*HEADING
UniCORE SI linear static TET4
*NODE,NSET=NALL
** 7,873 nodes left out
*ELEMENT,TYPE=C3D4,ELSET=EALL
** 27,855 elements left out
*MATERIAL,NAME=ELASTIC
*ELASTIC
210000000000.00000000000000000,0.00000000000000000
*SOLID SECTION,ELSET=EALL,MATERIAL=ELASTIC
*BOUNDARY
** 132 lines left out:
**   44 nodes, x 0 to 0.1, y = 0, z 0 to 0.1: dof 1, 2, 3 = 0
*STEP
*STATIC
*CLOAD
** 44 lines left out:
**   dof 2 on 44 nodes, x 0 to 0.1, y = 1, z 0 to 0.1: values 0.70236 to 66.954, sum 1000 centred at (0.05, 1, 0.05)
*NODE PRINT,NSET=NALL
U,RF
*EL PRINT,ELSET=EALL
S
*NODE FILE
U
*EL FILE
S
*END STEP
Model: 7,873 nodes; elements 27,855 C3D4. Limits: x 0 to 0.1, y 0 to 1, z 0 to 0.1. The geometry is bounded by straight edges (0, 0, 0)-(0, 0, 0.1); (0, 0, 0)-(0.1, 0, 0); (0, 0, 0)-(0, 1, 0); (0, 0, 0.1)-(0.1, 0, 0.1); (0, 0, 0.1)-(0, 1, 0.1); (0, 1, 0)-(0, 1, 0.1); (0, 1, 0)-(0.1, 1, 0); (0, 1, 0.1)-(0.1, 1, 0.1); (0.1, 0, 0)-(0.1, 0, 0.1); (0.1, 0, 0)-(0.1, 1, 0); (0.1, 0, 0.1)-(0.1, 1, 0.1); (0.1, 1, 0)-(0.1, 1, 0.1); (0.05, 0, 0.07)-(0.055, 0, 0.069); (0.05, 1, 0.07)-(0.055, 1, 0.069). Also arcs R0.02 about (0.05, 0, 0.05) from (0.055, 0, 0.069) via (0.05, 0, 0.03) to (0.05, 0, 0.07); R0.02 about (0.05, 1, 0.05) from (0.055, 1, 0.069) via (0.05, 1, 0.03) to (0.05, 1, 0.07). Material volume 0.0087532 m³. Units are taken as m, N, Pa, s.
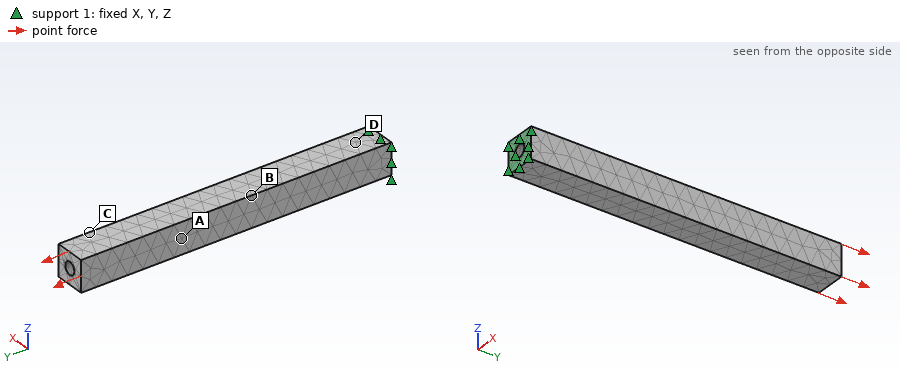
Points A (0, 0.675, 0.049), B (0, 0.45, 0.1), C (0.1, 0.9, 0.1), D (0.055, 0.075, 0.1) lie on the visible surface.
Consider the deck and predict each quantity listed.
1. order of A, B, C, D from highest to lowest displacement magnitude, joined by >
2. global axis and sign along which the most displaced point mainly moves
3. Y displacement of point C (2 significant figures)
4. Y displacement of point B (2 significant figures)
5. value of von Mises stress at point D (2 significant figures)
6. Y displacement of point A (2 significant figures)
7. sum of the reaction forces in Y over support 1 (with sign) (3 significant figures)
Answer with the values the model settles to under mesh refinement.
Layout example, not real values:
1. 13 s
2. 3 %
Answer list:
1. C > A > B > D
2. +Y
3. 4.9e-07 m
4. 2.4e-07 m
5. 1.1e+05 Pa
6. 3.7e-07 m
7. -1000 N
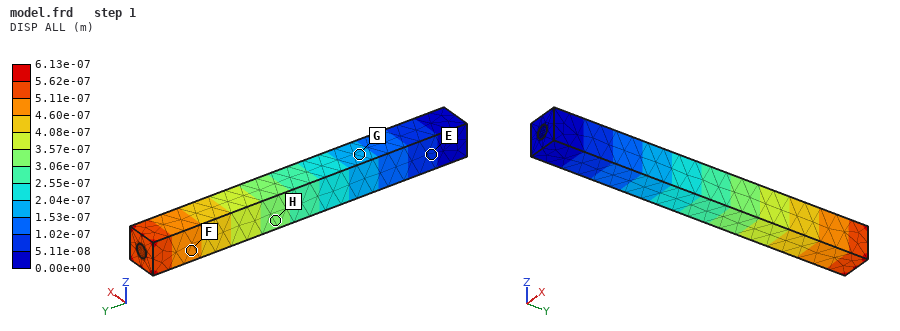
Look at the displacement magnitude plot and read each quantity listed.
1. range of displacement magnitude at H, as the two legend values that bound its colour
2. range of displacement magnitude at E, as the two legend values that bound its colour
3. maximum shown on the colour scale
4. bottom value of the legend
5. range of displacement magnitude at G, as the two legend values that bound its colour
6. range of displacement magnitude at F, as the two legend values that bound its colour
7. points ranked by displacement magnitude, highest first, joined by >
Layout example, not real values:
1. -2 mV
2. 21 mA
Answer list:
1. 3.06e-07 to 3.57e-07 m
2. 5.11e-08 to 1.02e-07 m
3. 6.13e-07 m
4. 0.00e+00 m
5. 1.53e-07 to 2.04e-07 m
6. 4.60e-07 to 5.11e-07 m
7. F > H > G > E
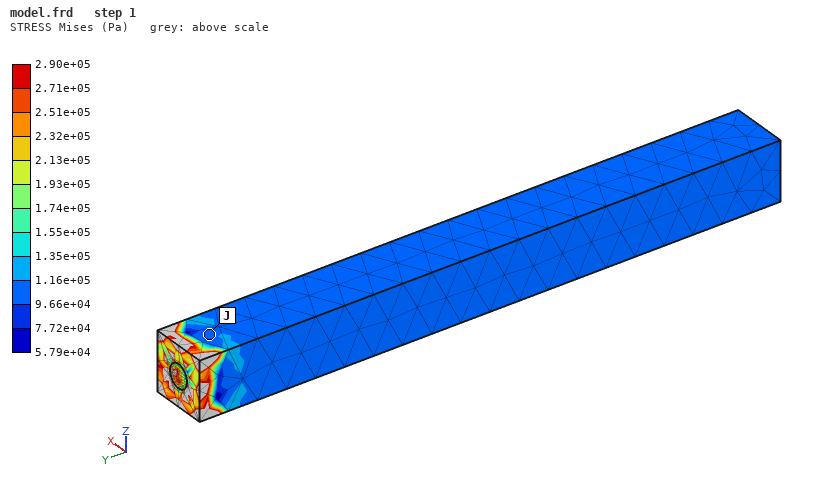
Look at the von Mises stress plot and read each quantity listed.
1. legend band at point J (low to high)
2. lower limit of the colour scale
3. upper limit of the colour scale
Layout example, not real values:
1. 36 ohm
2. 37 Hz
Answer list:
1. 9.66e+04 to 1.16e+05 Pa
2. 5.79e+04 Pa
3. 2.90e+05 Pa
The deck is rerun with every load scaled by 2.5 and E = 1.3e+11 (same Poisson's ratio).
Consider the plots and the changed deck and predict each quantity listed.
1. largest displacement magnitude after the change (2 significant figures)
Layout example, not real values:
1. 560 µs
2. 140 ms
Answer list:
1. 2.5e-06 m
